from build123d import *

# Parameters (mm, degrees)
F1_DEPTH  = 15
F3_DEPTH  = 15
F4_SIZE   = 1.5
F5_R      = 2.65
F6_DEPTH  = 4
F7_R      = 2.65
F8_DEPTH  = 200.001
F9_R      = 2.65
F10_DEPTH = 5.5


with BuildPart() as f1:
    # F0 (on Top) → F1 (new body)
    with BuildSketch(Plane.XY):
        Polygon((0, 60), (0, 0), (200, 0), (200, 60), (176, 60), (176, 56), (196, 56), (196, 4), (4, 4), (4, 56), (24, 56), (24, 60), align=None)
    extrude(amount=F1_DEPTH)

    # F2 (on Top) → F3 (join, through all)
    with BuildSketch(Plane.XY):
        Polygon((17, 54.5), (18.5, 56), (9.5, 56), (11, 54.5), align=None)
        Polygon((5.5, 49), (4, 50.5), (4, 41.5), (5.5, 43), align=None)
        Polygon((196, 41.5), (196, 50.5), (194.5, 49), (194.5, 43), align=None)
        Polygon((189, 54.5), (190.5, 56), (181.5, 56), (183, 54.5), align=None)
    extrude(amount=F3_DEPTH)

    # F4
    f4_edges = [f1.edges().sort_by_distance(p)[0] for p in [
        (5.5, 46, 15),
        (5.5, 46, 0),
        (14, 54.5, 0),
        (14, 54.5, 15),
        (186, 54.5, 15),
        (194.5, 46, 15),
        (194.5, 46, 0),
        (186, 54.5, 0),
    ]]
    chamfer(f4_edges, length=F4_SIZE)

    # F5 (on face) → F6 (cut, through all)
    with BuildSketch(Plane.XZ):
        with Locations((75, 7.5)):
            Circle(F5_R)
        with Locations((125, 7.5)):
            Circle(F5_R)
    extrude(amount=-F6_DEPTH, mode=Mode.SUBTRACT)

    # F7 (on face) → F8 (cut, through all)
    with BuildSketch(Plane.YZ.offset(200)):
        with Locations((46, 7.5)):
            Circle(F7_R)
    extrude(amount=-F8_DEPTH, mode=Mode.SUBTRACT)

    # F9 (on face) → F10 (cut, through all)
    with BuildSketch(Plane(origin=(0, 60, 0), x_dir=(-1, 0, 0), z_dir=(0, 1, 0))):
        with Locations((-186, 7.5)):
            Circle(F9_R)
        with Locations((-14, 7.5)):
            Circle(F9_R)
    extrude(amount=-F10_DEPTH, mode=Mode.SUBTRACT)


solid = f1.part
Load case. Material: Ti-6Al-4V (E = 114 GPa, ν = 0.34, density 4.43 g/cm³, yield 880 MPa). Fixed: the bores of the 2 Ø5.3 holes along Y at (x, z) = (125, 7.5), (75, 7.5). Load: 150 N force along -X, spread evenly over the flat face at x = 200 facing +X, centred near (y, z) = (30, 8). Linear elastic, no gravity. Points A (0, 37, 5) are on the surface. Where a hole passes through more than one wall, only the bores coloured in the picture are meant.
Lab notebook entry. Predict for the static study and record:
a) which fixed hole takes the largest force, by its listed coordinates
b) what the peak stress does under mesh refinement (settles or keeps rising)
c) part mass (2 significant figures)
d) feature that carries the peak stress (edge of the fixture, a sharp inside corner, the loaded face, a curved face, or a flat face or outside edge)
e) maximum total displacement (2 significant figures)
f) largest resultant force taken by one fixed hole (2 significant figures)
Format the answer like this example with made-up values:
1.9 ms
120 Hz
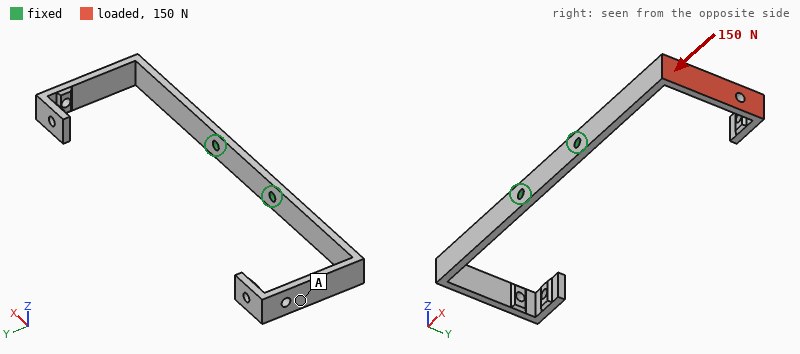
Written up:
(125, 7.5)
keeps rising
93 g
edge of the fixture
2.5 mm
150 N
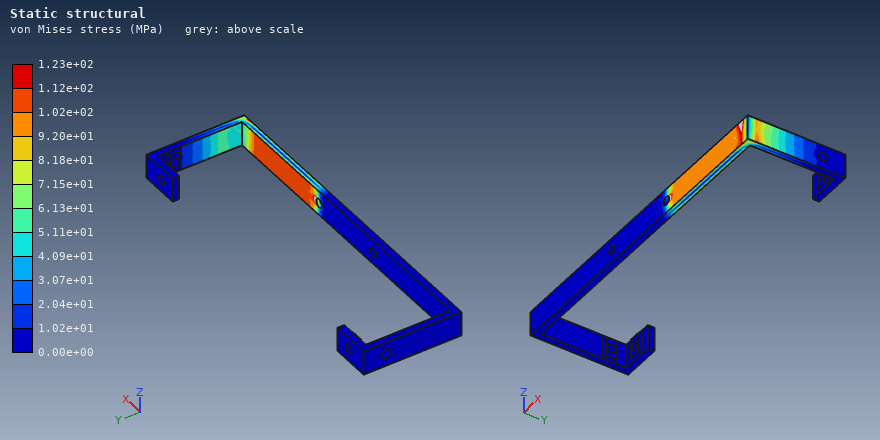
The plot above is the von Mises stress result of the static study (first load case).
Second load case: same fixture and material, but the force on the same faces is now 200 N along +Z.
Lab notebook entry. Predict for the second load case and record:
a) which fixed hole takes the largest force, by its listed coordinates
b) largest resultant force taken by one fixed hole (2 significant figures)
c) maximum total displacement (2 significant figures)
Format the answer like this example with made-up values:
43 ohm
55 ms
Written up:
(125, 7.5)
310 N
2.1 mm
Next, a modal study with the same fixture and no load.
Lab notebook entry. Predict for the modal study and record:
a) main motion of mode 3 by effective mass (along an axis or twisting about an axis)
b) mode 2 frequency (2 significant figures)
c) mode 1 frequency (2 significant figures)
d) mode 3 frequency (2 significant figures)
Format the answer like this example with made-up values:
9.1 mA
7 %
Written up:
along Z
210 Hz
210 Hz
340 Hz
